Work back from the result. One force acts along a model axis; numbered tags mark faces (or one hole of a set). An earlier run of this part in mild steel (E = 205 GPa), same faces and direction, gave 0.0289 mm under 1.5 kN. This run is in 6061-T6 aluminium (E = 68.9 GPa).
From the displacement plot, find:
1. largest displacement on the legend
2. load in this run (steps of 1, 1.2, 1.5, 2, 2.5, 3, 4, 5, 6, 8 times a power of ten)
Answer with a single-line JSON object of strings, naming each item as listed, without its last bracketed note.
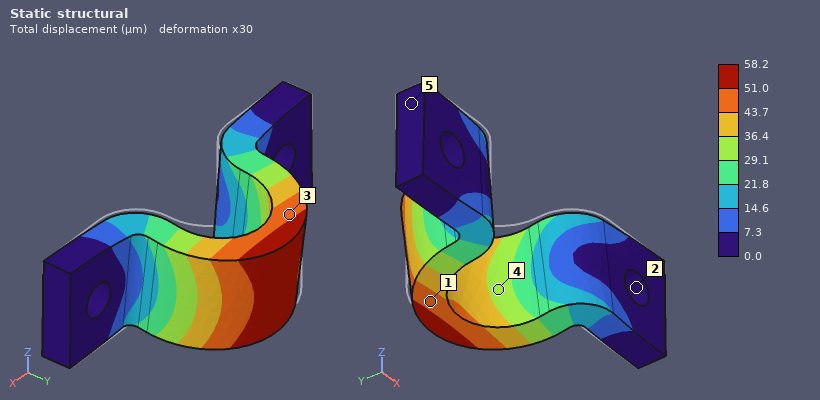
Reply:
{"largest displacement on the legend": "58.2 µm", "load in this run": "1 kN"}
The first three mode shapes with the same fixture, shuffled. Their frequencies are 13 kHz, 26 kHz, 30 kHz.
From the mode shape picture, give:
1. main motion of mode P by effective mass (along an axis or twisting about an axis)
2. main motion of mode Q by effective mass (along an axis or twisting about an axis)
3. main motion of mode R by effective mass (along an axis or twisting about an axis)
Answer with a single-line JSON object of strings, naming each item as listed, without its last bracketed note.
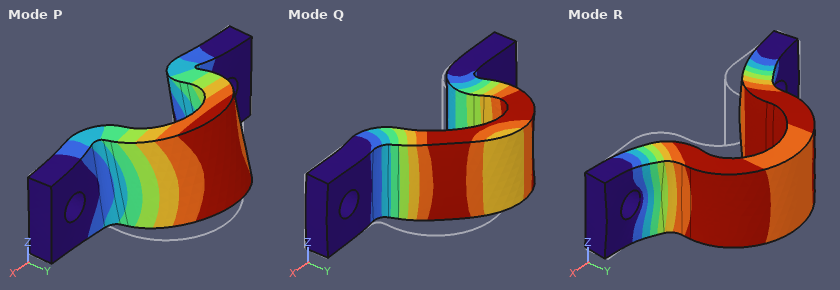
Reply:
{"main motion of mode P by effective mass": "along Z", "main motion of mode Q by effective mass": "along X", "main motion of mode R by effective mass": "along Y"}
